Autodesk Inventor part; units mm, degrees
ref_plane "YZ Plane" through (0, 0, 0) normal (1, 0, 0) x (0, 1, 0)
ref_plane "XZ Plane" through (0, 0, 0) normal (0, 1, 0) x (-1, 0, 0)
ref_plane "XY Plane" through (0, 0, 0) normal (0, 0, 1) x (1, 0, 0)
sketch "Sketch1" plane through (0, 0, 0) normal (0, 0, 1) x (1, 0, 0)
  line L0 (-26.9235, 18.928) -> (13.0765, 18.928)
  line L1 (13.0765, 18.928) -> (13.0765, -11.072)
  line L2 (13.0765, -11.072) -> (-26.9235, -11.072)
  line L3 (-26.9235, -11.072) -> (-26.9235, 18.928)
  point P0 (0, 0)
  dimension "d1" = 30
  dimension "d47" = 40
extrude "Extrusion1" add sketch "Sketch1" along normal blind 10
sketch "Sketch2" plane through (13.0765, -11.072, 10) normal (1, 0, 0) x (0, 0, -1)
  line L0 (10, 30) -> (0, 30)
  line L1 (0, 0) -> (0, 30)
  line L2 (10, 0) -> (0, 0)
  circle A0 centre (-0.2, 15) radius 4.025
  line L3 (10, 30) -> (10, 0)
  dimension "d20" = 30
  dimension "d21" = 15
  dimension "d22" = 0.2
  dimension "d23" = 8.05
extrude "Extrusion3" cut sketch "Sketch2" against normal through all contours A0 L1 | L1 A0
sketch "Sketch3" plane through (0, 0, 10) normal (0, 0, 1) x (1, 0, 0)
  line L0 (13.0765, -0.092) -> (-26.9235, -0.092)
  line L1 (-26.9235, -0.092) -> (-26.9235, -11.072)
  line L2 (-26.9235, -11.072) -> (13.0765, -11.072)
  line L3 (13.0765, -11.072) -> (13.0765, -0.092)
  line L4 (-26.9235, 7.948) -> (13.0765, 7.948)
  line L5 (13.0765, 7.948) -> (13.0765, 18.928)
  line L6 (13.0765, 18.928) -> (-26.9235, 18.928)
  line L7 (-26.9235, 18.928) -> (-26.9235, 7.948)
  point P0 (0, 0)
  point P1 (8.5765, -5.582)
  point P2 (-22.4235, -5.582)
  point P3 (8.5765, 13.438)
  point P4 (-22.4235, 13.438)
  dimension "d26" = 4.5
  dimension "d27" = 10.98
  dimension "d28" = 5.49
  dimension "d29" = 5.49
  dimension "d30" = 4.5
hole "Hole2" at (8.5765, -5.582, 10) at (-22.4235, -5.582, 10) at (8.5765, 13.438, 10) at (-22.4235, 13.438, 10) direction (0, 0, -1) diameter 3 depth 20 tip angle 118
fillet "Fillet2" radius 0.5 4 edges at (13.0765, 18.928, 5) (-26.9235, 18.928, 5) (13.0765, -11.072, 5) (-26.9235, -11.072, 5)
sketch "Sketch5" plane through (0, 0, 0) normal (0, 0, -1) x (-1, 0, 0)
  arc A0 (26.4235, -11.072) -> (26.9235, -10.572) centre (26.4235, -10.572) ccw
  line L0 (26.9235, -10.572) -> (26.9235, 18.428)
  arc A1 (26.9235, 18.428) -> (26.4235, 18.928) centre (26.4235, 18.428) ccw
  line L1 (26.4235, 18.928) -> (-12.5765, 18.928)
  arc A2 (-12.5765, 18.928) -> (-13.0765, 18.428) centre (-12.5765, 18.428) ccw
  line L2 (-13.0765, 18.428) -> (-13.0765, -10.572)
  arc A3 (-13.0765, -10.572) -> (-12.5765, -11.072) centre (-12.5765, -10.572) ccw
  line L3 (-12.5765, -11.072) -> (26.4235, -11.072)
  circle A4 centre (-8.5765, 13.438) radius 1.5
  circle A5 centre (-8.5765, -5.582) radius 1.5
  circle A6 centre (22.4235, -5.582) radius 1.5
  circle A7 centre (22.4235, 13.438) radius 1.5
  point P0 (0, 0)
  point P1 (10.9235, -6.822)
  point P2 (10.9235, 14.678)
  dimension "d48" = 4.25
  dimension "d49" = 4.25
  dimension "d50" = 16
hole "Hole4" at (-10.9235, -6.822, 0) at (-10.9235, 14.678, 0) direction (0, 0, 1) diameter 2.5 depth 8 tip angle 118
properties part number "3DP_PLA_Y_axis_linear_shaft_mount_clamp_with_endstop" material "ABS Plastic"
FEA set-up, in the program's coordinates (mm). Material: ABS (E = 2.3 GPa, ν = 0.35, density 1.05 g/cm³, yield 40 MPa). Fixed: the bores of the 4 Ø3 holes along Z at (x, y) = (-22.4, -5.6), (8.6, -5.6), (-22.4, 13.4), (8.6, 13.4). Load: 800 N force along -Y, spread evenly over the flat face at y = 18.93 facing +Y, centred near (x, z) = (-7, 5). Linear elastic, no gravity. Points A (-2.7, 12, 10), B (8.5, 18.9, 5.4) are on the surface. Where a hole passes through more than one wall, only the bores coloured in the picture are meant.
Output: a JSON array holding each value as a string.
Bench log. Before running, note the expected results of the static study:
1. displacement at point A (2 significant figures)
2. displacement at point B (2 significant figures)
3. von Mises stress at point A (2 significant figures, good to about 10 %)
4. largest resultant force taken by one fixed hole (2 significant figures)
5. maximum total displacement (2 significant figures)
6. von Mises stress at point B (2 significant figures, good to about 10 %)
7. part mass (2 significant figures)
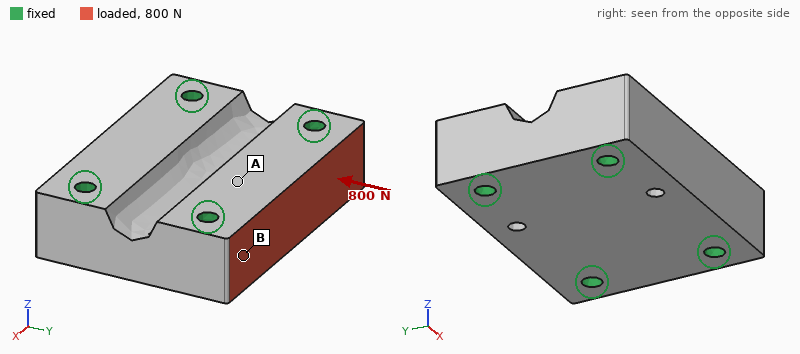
["23 µm", "6.7 µm", "1.4 MPa", "300 N", "30 µm", "3.3 MPa", "11 g"]
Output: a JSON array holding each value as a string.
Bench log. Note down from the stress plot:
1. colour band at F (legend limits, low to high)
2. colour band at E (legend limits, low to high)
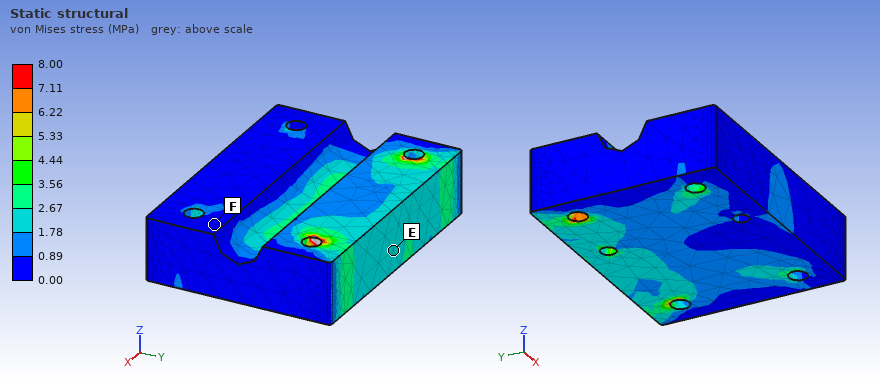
["0.00 to 0.89 MPa", "1.78 to 2.67 MPa"]
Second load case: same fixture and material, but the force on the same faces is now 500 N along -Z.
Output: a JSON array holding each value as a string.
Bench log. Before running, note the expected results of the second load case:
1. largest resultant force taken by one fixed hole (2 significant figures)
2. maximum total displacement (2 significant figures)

["270 N", "74 µm"]
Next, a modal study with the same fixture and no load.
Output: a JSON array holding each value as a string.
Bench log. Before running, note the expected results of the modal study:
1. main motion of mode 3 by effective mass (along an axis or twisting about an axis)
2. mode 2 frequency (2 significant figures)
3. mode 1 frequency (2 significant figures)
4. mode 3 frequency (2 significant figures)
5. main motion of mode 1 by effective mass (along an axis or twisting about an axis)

["along Y", "11 kHz", "9300 Hz", "12 kHz", "along Z"]
